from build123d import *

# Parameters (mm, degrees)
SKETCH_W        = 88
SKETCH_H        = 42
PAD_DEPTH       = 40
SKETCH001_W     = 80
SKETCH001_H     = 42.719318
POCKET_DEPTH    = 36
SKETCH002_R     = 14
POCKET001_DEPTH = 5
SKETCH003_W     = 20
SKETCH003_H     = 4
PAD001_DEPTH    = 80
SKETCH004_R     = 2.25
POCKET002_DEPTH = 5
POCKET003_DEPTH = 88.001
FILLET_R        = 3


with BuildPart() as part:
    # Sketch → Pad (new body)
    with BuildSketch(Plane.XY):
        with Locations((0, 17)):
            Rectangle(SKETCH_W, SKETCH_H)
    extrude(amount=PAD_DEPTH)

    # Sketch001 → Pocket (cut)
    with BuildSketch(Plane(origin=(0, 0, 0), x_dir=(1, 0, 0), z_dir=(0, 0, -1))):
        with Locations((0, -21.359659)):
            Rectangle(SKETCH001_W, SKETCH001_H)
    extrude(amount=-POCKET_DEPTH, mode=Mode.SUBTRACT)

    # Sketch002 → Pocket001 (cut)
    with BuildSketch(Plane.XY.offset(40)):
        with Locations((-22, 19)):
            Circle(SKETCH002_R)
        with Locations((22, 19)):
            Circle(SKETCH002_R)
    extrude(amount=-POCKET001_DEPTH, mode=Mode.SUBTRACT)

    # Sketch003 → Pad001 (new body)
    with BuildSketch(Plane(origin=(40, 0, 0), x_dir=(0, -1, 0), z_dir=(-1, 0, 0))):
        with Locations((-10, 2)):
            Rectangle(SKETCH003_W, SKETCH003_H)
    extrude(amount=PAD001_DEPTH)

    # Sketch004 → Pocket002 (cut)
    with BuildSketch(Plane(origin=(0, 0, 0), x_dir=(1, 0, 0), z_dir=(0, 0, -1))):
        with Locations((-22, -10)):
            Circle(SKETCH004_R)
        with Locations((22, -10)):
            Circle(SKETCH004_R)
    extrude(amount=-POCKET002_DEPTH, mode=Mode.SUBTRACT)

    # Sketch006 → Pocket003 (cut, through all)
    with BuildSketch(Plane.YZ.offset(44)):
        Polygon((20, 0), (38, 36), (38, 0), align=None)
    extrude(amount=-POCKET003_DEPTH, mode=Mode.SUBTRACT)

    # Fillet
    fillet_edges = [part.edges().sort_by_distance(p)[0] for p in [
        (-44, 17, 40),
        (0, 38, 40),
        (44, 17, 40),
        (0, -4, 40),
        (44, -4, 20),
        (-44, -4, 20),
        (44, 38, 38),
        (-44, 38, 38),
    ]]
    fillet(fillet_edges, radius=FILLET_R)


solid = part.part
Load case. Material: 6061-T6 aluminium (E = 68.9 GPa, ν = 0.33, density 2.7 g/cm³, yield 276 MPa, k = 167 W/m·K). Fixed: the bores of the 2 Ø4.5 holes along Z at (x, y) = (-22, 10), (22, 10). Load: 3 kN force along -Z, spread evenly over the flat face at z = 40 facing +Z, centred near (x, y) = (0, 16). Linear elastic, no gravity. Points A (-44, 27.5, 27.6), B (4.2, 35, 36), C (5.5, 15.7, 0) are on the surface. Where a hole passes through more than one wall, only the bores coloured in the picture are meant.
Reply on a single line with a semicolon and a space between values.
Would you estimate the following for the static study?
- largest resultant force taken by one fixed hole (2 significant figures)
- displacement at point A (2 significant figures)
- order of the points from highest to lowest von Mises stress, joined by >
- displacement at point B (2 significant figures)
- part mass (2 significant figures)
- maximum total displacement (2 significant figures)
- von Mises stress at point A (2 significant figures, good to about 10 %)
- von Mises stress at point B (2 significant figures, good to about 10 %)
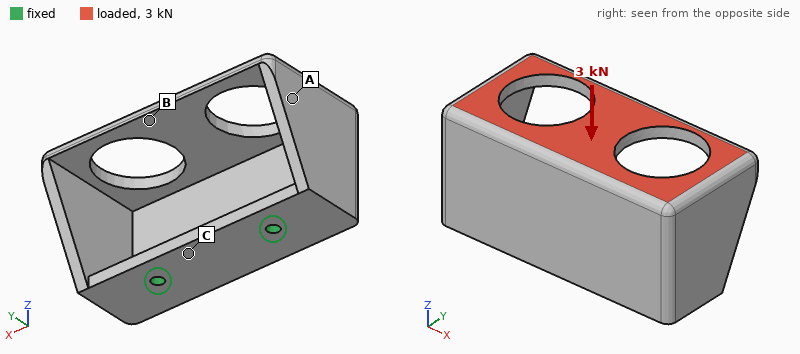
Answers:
1.5 kN; 0.47 mm; B > A > C; 1.0 mm; 99 g; 1.1 mm; 50 MPa; 100 MPa
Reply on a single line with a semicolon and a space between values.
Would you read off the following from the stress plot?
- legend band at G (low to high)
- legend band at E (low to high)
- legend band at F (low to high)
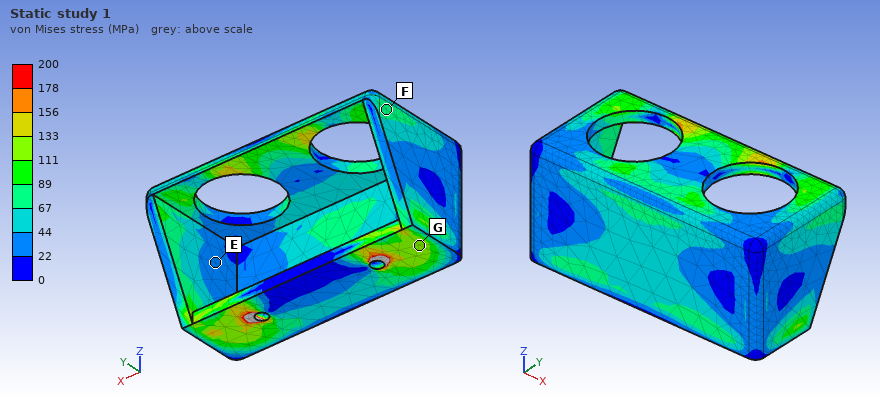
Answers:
111 to 133 MPa; 22 to 44 MPa; 67 to 89 MPa
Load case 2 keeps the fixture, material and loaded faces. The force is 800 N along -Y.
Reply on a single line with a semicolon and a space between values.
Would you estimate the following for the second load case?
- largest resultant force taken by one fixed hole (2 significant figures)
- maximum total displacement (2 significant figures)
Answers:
430 N; 0.60 mm
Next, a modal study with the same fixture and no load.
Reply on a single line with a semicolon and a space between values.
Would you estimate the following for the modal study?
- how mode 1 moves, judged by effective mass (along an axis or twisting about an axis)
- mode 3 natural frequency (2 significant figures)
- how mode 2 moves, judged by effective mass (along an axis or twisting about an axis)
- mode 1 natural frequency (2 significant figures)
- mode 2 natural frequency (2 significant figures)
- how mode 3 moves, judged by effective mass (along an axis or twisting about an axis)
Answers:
along Y; 3000 Hz; along X; 990 Hz; 1500 Hz; along Z
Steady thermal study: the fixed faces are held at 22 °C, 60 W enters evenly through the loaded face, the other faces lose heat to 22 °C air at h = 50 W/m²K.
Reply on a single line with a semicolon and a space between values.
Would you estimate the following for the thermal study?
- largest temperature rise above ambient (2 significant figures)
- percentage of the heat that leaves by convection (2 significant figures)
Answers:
53 K; 33 %
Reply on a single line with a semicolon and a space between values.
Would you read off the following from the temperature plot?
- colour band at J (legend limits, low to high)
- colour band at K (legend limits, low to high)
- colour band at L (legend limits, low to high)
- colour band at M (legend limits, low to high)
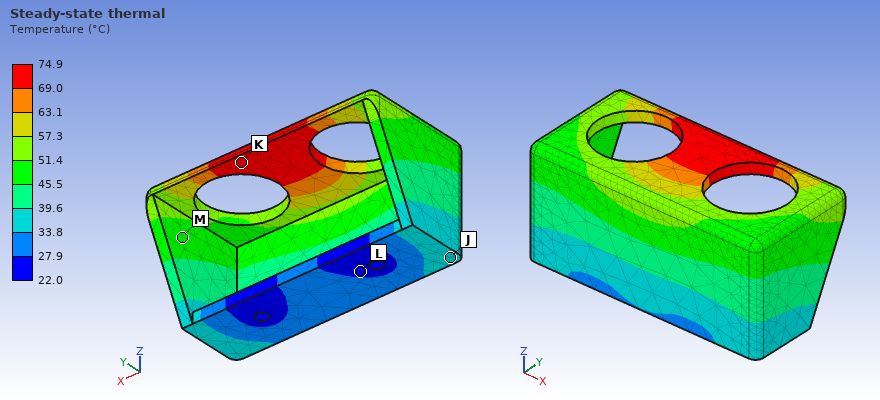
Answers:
33.8 to 39.6 °C; 69.0 to 74.9 °C; 22.0 to 27.9 °C; 45.5 to 51.4 °C
